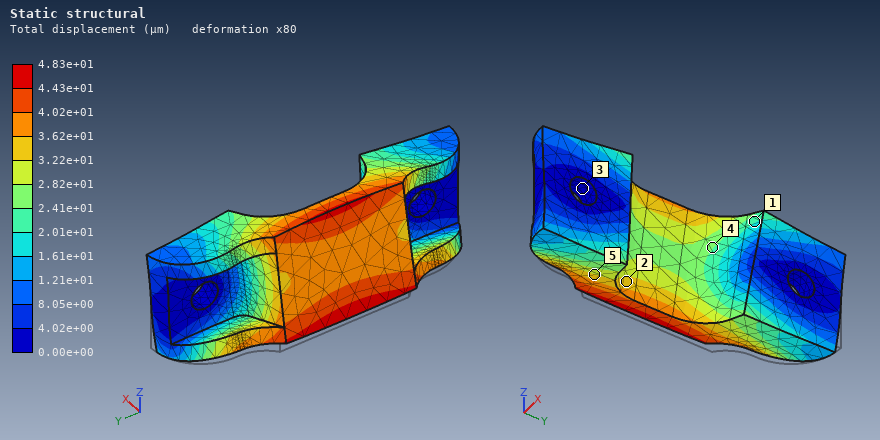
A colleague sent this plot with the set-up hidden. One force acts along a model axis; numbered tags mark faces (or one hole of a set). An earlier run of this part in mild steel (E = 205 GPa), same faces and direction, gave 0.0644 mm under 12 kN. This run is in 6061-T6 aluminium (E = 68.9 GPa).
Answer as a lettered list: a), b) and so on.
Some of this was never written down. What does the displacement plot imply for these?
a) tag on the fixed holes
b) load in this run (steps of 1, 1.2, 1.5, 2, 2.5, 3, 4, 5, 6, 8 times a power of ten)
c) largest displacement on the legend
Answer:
a) 3
b) 3 kN
c) 4.83e+01 µm
